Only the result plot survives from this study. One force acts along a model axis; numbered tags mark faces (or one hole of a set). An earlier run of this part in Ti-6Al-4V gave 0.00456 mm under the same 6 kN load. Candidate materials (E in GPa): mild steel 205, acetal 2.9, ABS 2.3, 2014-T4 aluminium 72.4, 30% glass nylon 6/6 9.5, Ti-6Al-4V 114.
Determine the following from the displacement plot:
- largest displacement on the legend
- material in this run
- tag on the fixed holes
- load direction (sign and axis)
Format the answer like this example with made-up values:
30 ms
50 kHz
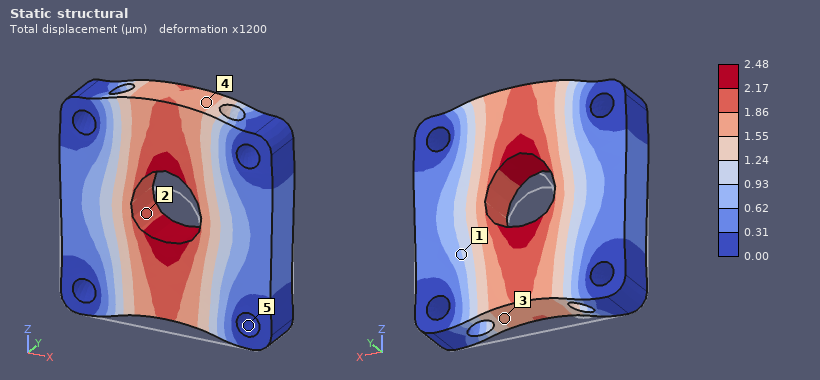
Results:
2.48 µm
mild steel
5
+Z
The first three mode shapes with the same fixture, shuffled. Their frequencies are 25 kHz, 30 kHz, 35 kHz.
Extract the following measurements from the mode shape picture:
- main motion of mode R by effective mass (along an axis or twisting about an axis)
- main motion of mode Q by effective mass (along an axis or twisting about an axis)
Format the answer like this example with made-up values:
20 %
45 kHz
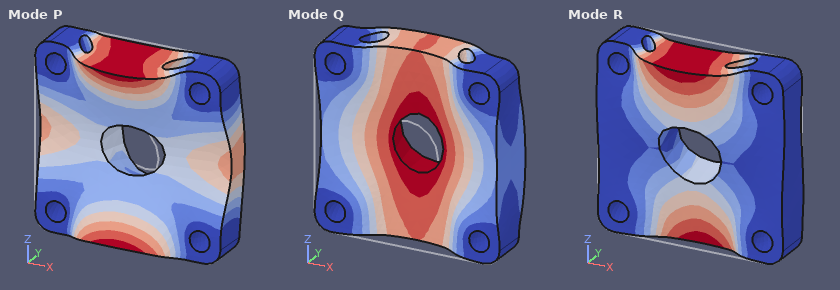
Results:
twisting about X
along Y
